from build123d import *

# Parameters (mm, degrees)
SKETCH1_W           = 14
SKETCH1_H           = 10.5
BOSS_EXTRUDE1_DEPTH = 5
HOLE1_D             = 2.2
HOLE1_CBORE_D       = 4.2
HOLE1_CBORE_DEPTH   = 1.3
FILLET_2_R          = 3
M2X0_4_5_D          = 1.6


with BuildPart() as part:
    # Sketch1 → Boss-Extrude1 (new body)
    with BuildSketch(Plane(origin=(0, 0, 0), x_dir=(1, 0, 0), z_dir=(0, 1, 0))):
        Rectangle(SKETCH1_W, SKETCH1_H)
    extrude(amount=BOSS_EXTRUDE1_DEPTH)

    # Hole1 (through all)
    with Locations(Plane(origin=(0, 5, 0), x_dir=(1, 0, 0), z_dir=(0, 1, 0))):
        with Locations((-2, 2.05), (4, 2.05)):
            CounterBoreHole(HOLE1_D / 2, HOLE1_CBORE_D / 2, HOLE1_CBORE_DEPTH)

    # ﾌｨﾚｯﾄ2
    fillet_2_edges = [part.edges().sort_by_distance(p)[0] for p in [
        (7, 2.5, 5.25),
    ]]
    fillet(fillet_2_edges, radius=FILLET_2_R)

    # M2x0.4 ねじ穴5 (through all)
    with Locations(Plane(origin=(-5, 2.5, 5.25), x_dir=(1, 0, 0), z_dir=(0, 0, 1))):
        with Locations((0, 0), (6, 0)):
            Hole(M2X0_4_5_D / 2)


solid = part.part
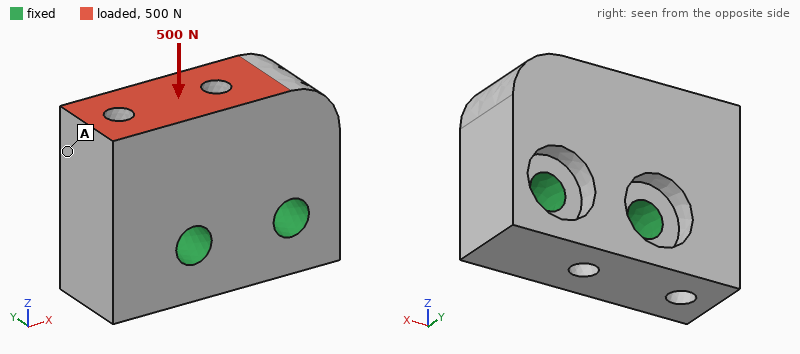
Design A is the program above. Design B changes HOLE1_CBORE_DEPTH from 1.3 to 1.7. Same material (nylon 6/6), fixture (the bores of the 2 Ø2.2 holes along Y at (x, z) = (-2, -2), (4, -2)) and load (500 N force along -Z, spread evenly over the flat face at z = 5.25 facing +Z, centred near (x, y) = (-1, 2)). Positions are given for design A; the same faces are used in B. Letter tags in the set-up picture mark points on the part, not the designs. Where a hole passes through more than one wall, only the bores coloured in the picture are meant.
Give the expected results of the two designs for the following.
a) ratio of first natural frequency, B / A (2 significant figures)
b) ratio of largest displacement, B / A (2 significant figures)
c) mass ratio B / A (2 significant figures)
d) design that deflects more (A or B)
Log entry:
0.90
1.2
0.99
B
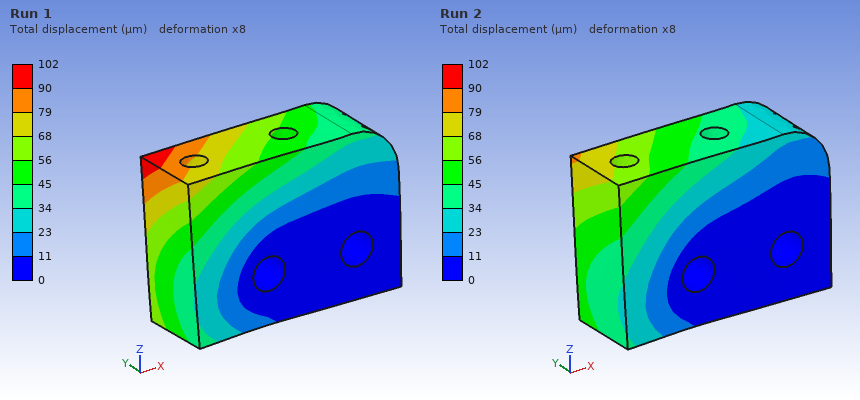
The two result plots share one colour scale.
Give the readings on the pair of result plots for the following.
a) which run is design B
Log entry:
Run 1
